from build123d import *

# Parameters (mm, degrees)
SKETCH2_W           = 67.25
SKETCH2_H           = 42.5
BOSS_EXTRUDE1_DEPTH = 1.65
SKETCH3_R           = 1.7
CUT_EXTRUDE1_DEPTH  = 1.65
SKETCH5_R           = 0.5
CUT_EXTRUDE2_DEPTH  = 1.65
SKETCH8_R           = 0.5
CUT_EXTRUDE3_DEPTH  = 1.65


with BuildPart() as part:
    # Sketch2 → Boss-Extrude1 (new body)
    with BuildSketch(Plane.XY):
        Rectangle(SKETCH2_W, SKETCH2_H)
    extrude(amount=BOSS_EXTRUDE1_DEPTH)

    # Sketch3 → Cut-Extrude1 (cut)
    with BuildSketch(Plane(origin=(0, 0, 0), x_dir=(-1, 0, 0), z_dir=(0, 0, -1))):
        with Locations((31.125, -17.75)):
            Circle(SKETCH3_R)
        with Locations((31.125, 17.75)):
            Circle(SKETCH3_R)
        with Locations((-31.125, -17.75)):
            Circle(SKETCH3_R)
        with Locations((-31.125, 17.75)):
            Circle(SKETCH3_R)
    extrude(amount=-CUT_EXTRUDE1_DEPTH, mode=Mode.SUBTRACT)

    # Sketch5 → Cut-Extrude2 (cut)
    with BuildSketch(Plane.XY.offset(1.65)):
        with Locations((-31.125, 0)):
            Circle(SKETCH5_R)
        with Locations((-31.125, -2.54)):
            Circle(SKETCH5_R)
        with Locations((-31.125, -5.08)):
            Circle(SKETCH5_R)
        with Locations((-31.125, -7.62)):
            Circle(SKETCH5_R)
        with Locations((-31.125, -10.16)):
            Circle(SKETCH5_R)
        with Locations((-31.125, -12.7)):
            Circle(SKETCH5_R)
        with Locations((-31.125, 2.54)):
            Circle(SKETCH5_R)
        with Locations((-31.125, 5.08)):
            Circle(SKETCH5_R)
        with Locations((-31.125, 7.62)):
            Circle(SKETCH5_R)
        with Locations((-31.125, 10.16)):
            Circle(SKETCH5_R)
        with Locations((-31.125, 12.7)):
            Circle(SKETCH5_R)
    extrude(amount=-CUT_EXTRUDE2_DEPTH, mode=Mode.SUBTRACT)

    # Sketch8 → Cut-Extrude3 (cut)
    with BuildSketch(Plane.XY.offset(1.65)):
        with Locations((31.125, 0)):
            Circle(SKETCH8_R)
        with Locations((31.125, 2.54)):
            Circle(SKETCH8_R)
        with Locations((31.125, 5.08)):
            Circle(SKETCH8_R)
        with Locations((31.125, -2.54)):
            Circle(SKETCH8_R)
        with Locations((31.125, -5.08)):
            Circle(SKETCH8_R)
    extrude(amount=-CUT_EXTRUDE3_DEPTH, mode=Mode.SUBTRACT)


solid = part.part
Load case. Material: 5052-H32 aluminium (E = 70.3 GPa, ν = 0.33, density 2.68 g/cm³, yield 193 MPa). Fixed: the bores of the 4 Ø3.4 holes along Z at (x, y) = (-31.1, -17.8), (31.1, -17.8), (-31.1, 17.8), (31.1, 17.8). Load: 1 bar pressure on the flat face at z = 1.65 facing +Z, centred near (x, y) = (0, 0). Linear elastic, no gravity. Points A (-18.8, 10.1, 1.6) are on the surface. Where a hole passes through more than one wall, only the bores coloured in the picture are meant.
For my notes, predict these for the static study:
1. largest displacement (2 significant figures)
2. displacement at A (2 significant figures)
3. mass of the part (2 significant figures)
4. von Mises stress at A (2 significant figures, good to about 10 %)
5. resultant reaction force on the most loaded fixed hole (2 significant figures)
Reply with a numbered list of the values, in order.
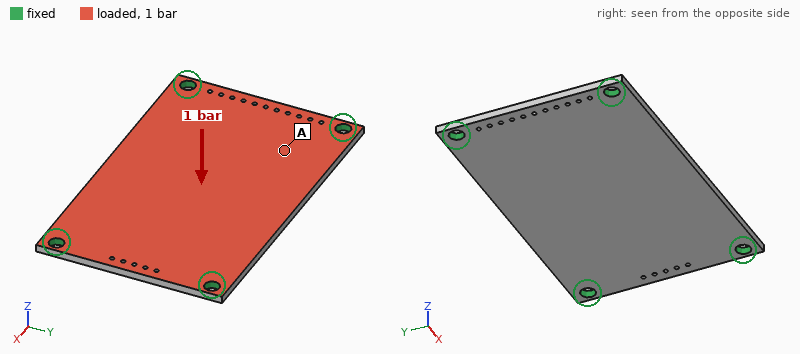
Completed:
1. 0.19 mm
2. 0.089 mm
3. 12 g
4. 11 MPa
5. 70 N
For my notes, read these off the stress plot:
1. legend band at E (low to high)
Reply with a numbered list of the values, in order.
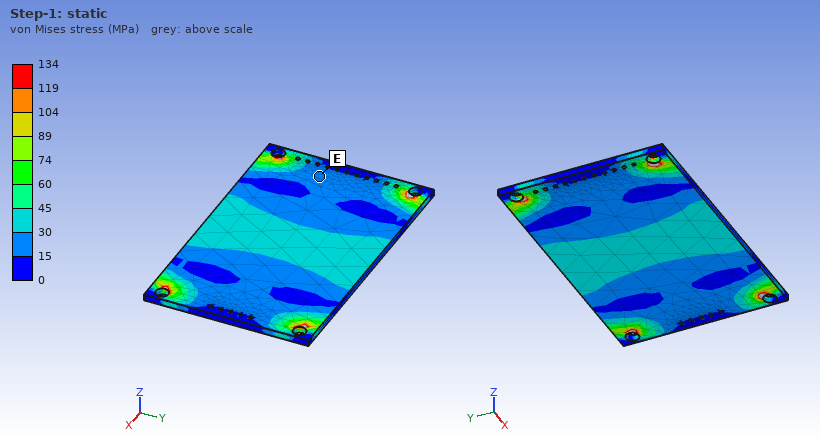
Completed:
1. 15 to 30 MPa
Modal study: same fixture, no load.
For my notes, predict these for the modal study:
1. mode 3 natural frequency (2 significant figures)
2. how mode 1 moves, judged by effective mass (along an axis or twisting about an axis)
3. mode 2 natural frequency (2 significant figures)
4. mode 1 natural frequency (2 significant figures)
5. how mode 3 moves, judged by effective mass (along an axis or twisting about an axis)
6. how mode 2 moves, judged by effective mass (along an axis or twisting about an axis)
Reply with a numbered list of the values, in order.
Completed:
1. 5300 Hz
2. along Z
3. 3300 Hz
4. 2000 Hz
5. twisting about Y
6. twisting about X
